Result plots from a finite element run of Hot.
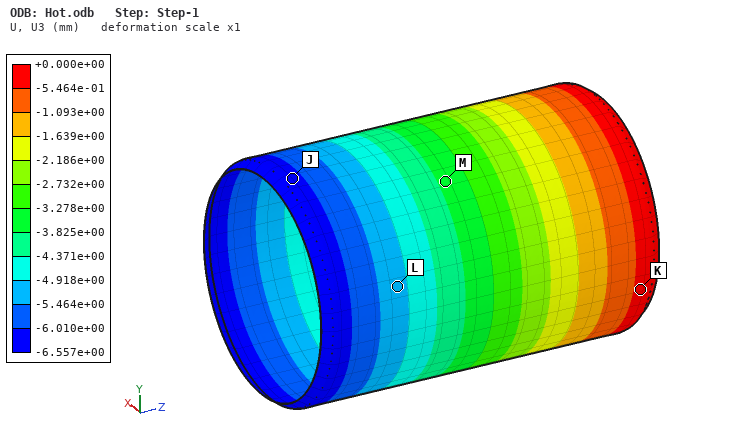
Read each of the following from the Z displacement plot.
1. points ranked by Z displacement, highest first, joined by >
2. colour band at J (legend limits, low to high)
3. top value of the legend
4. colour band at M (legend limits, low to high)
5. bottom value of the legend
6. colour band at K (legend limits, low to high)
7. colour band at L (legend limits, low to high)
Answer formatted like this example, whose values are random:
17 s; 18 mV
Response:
K > M > L > J; -6.557e+00 to -6.010e+00 mm; +0.000e+00 mm; -3.825e+00 to -3.278e+00 mm; -6.557e+00 mm; -5.464e-01 to +0.000e+00 mm; -5.464e+00 to -4.918e+00 mm
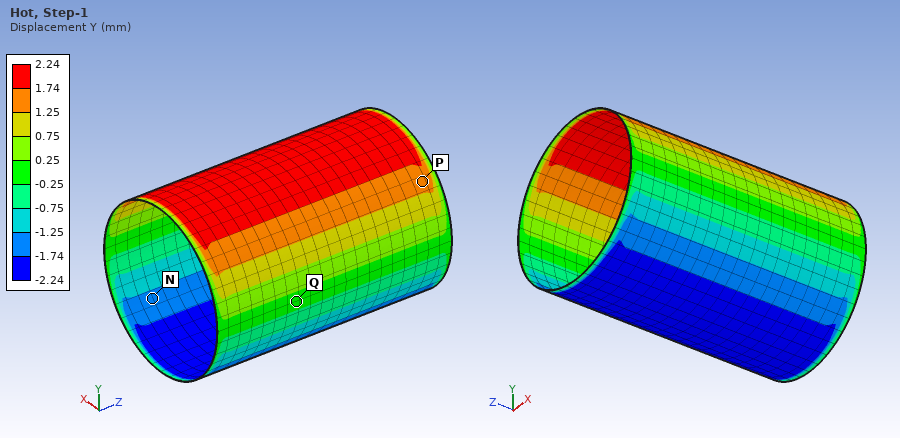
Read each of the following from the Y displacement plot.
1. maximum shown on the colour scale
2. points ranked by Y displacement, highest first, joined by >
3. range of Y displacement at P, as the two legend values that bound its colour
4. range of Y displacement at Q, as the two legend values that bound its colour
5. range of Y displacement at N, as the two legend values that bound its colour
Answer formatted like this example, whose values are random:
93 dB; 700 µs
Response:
2.24 mm; P > Q > N; 1.25 to 1.74 mm; -0.25 to 0.25 mm; -1.74 to -1.25 mm
